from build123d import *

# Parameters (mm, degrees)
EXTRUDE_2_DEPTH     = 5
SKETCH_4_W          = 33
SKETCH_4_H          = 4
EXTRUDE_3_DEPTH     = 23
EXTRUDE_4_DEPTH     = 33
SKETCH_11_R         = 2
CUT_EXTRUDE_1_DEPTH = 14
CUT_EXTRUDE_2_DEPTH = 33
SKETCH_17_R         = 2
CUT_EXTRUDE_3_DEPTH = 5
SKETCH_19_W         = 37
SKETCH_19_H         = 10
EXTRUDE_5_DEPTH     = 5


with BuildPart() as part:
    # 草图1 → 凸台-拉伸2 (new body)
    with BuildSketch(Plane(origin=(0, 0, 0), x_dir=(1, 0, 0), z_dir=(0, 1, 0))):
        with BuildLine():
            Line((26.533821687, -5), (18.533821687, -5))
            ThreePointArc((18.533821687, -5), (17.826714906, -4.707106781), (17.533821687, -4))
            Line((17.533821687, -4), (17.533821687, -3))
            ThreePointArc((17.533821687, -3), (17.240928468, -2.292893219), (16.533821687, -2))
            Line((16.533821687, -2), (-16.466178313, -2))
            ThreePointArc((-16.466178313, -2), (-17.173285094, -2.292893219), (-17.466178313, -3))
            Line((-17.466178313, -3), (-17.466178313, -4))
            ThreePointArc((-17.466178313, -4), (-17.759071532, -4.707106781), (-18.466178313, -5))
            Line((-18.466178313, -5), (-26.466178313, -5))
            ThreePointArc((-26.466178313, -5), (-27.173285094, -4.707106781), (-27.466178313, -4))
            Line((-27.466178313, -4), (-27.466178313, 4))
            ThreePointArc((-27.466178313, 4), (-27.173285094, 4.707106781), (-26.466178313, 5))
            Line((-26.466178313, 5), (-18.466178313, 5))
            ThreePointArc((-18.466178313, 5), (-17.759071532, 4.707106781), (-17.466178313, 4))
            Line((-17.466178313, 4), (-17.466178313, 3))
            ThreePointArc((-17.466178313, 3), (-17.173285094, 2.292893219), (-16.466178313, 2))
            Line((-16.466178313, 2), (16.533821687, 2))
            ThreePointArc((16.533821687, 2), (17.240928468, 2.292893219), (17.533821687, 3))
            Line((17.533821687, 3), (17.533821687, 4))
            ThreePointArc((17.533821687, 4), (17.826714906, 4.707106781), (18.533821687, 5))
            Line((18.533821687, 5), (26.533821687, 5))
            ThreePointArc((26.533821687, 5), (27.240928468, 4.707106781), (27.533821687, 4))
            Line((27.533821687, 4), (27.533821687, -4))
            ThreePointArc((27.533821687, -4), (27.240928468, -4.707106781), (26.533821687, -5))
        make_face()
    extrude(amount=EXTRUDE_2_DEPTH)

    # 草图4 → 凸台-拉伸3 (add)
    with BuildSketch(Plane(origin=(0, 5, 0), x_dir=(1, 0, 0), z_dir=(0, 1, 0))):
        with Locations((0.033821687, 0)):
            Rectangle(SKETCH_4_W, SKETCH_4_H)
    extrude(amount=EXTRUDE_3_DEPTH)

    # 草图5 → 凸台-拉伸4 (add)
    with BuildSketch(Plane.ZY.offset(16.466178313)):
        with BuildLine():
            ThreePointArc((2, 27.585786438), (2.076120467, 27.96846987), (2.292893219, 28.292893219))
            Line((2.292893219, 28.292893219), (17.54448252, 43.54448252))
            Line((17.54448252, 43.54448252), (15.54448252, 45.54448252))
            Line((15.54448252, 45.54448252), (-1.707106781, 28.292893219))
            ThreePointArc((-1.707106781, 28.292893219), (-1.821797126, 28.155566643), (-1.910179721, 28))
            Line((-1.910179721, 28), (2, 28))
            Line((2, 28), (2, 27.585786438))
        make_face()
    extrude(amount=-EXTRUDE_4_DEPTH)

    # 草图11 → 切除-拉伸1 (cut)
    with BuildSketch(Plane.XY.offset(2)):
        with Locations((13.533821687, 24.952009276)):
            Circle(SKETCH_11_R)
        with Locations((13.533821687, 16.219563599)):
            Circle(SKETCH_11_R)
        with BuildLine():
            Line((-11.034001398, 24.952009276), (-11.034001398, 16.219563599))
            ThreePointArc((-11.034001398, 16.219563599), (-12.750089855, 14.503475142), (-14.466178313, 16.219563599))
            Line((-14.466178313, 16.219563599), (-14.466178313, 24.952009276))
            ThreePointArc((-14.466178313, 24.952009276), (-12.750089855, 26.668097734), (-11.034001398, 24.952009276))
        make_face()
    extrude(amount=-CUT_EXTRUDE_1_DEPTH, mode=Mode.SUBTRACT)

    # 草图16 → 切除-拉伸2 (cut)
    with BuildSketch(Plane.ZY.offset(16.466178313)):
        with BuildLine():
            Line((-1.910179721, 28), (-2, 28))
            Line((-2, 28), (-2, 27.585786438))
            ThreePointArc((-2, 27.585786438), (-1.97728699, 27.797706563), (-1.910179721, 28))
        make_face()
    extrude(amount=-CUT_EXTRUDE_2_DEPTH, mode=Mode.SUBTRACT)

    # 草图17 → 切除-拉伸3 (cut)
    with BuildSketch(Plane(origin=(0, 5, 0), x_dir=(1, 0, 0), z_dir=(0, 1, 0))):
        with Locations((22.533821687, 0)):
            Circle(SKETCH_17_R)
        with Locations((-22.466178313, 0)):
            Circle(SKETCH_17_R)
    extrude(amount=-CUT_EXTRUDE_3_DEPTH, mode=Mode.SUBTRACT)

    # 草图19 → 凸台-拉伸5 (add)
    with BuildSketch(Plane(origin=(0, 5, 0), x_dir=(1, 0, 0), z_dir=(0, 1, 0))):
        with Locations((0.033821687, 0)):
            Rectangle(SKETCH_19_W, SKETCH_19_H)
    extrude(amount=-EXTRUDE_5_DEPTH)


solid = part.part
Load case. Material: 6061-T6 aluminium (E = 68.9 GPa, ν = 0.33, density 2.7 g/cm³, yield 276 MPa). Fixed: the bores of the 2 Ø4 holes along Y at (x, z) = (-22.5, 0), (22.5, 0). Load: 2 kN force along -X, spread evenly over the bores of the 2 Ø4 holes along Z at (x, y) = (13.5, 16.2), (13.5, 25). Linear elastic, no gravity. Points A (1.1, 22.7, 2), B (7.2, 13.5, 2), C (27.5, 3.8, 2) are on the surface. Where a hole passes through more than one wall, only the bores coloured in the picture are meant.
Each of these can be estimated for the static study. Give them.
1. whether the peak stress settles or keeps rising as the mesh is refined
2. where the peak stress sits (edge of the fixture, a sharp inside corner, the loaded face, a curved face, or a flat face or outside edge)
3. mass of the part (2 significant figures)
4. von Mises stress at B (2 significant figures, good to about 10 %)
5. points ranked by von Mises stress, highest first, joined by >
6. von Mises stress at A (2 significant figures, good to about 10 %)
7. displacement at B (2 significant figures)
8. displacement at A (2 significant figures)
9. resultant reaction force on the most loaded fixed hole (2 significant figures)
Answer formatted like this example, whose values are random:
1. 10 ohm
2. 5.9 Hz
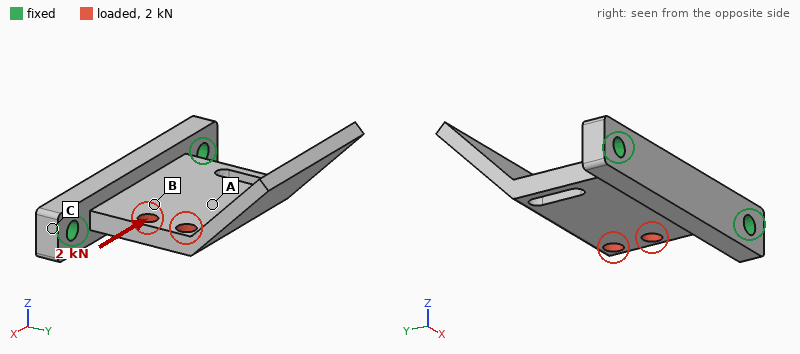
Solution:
1. keeps rising
2. edge of the fixture
3. 20 g
4. 33 MPa
5. B > A > C
6. 22 MPa
7. 18 µm
8. 30 µm
9. 1.4 kN
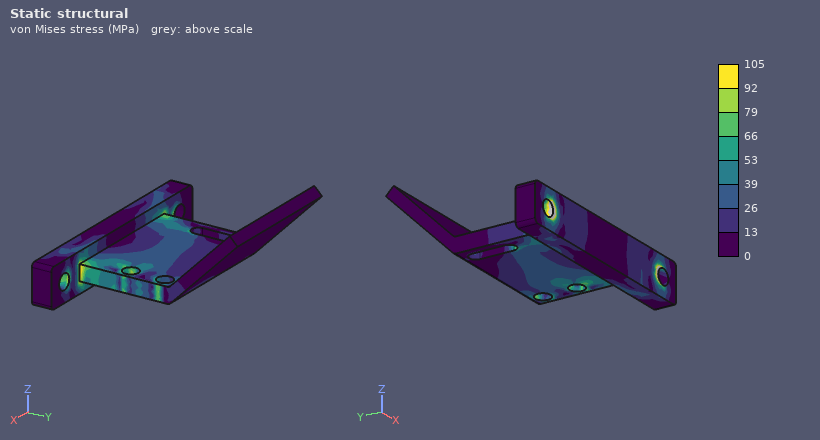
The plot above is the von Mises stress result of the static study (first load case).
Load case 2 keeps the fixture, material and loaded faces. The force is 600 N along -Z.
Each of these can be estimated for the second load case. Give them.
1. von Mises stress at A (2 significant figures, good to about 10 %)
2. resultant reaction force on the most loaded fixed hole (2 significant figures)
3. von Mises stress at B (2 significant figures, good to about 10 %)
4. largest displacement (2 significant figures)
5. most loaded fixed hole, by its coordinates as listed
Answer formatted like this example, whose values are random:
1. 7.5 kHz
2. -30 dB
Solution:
1. 40 MPa
2. 520 N
3. 83 MPa
4. 0.66 mm
5. (22.5, 0)
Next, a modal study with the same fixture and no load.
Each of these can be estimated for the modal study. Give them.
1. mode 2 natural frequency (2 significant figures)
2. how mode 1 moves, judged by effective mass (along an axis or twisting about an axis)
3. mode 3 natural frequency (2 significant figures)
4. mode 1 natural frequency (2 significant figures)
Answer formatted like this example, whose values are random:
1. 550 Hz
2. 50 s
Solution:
1. 3700 Hz
2. along Z
3. 5300 Hz
4. 1400 Hz
